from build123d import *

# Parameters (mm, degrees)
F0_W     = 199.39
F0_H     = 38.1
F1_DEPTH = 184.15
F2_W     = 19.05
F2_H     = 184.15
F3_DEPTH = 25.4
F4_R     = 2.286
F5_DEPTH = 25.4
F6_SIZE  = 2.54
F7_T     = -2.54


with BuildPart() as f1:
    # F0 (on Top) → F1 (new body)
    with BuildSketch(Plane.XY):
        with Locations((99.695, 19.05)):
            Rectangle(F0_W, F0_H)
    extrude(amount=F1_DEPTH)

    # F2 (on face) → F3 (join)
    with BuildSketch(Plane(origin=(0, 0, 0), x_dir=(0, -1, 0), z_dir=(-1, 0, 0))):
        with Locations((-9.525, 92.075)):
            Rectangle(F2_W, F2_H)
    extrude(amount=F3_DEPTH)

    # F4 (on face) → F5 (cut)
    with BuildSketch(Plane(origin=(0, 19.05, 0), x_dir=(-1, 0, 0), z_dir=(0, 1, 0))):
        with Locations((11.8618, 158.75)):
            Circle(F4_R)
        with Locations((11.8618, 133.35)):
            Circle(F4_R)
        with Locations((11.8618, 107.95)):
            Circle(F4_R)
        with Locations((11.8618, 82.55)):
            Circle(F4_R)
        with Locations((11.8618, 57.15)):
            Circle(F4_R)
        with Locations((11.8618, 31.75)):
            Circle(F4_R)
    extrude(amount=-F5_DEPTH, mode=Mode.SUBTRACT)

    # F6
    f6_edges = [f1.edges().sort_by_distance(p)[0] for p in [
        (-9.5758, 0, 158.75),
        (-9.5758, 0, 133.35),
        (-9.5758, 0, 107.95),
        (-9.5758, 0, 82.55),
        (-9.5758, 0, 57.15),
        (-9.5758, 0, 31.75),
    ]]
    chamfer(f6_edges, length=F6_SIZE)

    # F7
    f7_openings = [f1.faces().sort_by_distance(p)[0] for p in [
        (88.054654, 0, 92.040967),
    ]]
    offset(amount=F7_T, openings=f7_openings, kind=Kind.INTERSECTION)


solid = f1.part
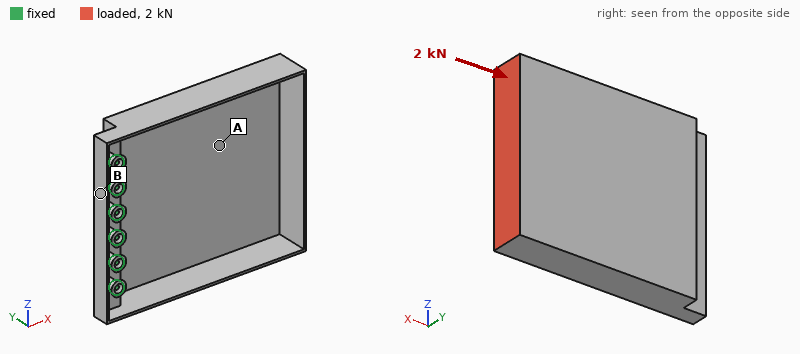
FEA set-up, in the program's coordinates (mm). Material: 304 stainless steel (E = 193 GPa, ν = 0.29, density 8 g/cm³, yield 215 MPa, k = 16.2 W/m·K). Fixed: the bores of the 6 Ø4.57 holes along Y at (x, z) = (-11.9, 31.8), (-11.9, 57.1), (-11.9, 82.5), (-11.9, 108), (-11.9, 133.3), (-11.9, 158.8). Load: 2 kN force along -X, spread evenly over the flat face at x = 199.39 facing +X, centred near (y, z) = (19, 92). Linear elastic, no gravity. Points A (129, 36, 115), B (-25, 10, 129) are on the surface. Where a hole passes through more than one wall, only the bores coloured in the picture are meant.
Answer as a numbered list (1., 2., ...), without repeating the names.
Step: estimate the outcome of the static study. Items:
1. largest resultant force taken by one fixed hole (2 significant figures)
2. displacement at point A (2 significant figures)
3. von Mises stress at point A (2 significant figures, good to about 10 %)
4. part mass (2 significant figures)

1. 1.5 kN
2. 0.20 mm
3. 18 MPa
4. 1.5 kg
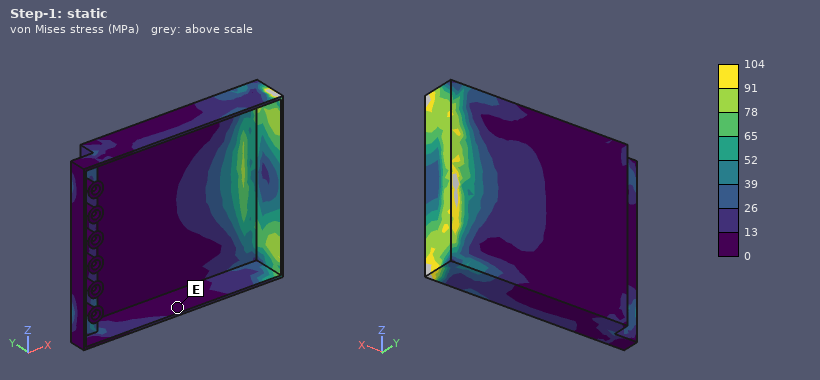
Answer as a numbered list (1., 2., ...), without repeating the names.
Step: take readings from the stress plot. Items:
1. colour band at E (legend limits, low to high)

1. 0 to 13 MPa
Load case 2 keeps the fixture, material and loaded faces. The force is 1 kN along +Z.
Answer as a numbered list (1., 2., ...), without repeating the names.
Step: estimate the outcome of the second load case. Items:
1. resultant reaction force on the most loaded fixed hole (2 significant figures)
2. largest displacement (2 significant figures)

1. 2.4 kN
2. 2.7 mm
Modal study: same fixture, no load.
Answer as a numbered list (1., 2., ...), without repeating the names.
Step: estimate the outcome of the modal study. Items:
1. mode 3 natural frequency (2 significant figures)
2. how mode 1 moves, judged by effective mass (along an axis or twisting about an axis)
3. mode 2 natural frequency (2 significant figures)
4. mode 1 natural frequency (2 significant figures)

1. 490 Hz
2. along Y
3. 130 Hz
4. 92 Hz
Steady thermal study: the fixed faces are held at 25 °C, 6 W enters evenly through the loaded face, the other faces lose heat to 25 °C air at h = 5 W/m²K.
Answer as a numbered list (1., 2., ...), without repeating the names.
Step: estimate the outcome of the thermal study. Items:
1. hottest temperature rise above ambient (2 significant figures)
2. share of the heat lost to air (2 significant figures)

1. 41 K
2. 96 %
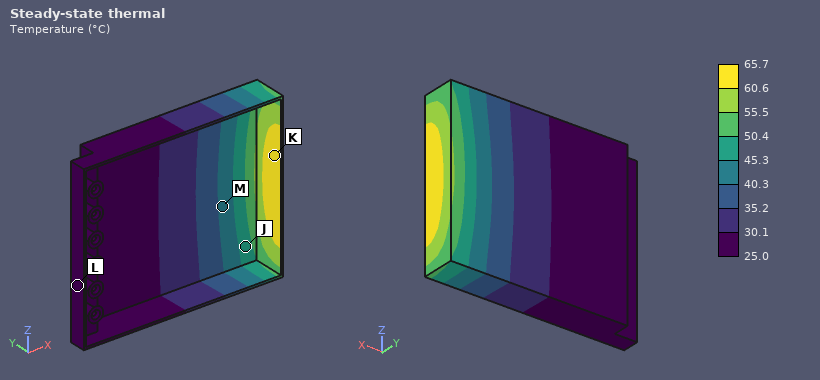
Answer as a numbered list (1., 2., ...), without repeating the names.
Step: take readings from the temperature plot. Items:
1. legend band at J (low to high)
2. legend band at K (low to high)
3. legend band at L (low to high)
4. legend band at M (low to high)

1. 45.3 to 50.4 °C
2. 60.6 to 65.7 °C
3. 25.0 to 30.1 °C
4. 40.3 to 45.3 °C
